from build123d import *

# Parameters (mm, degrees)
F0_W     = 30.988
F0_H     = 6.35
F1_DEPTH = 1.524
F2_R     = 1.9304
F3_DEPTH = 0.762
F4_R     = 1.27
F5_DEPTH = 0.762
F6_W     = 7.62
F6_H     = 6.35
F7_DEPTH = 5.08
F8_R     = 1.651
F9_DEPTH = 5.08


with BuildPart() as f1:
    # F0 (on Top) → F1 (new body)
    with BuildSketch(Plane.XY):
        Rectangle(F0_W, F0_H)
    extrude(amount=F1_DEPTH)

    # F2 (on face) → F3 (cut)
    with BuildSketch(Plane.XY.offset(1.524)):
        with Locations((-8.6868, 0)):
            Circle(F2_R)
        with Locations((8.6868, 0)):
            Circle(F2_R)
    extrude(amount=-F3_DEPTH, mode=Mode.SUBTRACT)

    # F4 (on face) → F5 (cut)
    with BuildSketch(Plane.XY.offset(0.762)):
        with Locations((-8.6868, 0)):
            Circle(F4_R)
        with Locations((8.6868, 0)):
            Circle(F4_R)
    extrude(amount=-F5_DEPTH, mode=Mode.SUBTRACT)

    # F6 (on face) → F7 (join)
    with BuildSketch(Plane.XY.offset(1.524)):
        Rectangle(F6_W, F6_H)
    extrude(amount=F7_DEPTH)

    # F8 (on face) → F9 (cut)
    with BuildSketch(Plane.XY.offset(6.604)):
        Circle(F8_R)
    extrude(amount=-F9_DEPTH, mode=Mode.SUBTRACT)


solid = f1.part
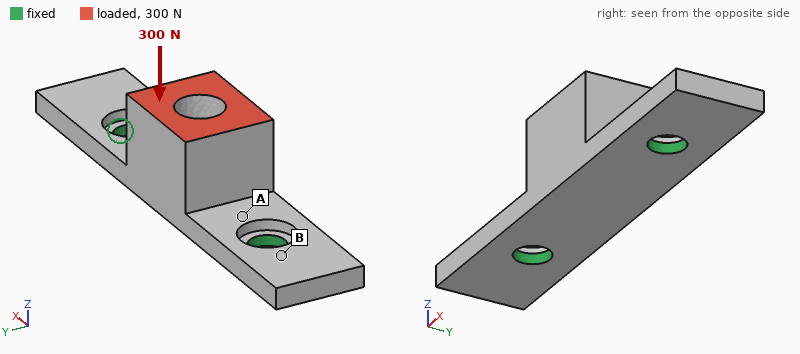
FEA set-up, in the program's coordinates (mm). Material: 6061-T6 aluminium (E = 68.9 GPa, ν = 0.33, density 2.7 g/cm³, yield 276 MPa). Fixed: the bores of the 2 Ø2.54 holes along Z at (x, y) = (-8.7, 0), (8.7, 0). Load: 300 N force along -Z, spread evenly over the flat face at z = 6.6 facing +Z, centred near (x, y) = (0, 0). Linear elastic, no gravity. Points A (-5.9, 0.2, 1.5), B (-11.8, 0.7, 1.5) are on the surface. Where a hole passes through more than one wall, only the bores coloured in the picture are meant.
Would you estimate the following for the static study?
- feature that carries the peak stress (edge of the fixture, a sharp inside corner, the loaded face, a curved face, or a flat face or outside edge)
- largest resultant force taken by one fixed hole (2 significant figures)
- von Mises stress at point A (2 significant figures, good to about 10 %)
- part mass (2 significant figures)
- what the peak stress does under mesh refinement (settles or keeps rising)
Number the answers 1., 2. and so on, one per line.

1. edge of the fixture
2. 240 N
3. 63 MPa
4. 1.3 g
5. keeps rising
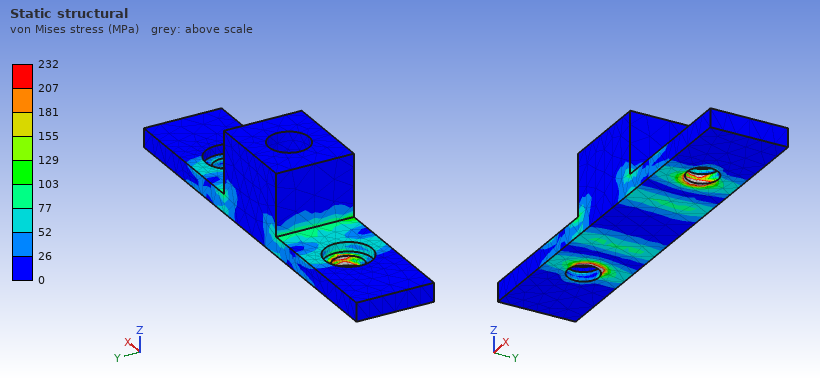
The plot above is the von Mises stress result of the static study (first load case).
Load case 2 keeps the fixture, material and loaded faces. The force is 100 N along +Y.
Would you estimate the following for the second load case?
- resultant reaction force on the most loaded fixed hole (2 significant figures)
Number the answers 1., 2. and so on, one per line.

1. 50 N
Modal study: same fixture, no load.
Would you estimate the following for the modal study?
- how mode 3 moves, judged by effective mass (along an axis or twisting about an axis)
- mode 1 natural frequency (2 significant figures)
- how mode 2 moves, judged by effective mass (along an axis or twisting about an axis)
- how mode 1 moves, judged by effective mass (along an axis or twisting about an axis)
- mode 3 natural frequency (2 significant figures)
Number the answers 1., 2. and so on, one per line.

1. twisting about Y
2. 12 kHz
3. along Z
4. along Y
5. 22 kHz
